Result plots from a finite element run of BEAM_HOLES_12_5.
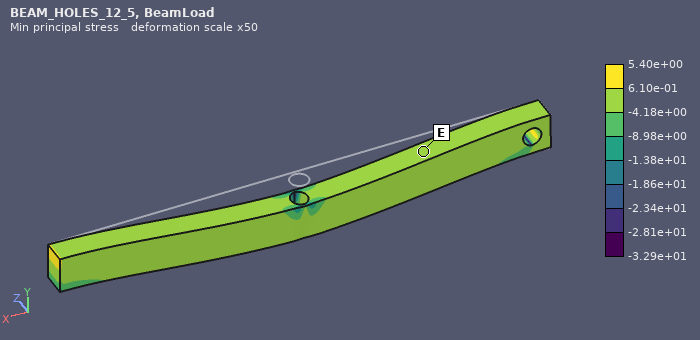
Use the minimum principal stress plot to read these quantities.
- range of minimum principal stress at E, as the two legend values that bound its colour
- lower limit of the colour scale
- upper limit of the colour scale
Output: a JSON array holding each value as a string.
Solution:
["-4.18e+00 to 6.10e-01", "-3.29e+01", "5.40e+00"]
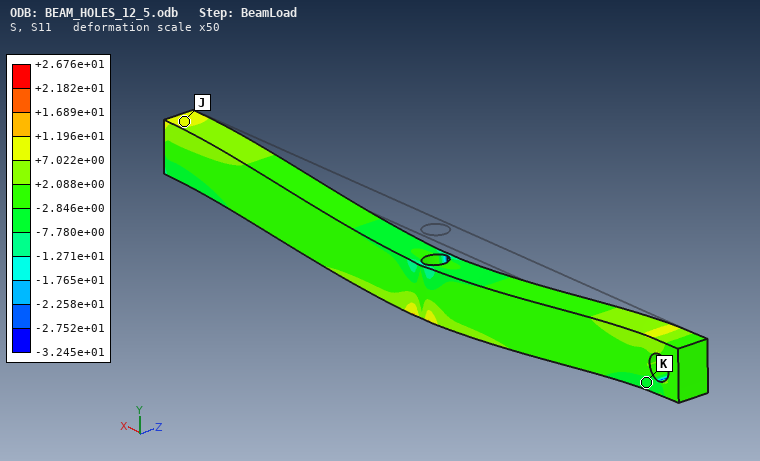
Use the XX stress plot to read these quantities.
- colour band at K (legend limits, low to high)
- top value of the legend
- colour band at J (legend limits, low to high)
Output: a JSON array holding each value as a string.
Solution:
["-7.780e+00 to -2.846e+00", "+2.676e+01", "+7.022e+00 to +1.196e+01"]
